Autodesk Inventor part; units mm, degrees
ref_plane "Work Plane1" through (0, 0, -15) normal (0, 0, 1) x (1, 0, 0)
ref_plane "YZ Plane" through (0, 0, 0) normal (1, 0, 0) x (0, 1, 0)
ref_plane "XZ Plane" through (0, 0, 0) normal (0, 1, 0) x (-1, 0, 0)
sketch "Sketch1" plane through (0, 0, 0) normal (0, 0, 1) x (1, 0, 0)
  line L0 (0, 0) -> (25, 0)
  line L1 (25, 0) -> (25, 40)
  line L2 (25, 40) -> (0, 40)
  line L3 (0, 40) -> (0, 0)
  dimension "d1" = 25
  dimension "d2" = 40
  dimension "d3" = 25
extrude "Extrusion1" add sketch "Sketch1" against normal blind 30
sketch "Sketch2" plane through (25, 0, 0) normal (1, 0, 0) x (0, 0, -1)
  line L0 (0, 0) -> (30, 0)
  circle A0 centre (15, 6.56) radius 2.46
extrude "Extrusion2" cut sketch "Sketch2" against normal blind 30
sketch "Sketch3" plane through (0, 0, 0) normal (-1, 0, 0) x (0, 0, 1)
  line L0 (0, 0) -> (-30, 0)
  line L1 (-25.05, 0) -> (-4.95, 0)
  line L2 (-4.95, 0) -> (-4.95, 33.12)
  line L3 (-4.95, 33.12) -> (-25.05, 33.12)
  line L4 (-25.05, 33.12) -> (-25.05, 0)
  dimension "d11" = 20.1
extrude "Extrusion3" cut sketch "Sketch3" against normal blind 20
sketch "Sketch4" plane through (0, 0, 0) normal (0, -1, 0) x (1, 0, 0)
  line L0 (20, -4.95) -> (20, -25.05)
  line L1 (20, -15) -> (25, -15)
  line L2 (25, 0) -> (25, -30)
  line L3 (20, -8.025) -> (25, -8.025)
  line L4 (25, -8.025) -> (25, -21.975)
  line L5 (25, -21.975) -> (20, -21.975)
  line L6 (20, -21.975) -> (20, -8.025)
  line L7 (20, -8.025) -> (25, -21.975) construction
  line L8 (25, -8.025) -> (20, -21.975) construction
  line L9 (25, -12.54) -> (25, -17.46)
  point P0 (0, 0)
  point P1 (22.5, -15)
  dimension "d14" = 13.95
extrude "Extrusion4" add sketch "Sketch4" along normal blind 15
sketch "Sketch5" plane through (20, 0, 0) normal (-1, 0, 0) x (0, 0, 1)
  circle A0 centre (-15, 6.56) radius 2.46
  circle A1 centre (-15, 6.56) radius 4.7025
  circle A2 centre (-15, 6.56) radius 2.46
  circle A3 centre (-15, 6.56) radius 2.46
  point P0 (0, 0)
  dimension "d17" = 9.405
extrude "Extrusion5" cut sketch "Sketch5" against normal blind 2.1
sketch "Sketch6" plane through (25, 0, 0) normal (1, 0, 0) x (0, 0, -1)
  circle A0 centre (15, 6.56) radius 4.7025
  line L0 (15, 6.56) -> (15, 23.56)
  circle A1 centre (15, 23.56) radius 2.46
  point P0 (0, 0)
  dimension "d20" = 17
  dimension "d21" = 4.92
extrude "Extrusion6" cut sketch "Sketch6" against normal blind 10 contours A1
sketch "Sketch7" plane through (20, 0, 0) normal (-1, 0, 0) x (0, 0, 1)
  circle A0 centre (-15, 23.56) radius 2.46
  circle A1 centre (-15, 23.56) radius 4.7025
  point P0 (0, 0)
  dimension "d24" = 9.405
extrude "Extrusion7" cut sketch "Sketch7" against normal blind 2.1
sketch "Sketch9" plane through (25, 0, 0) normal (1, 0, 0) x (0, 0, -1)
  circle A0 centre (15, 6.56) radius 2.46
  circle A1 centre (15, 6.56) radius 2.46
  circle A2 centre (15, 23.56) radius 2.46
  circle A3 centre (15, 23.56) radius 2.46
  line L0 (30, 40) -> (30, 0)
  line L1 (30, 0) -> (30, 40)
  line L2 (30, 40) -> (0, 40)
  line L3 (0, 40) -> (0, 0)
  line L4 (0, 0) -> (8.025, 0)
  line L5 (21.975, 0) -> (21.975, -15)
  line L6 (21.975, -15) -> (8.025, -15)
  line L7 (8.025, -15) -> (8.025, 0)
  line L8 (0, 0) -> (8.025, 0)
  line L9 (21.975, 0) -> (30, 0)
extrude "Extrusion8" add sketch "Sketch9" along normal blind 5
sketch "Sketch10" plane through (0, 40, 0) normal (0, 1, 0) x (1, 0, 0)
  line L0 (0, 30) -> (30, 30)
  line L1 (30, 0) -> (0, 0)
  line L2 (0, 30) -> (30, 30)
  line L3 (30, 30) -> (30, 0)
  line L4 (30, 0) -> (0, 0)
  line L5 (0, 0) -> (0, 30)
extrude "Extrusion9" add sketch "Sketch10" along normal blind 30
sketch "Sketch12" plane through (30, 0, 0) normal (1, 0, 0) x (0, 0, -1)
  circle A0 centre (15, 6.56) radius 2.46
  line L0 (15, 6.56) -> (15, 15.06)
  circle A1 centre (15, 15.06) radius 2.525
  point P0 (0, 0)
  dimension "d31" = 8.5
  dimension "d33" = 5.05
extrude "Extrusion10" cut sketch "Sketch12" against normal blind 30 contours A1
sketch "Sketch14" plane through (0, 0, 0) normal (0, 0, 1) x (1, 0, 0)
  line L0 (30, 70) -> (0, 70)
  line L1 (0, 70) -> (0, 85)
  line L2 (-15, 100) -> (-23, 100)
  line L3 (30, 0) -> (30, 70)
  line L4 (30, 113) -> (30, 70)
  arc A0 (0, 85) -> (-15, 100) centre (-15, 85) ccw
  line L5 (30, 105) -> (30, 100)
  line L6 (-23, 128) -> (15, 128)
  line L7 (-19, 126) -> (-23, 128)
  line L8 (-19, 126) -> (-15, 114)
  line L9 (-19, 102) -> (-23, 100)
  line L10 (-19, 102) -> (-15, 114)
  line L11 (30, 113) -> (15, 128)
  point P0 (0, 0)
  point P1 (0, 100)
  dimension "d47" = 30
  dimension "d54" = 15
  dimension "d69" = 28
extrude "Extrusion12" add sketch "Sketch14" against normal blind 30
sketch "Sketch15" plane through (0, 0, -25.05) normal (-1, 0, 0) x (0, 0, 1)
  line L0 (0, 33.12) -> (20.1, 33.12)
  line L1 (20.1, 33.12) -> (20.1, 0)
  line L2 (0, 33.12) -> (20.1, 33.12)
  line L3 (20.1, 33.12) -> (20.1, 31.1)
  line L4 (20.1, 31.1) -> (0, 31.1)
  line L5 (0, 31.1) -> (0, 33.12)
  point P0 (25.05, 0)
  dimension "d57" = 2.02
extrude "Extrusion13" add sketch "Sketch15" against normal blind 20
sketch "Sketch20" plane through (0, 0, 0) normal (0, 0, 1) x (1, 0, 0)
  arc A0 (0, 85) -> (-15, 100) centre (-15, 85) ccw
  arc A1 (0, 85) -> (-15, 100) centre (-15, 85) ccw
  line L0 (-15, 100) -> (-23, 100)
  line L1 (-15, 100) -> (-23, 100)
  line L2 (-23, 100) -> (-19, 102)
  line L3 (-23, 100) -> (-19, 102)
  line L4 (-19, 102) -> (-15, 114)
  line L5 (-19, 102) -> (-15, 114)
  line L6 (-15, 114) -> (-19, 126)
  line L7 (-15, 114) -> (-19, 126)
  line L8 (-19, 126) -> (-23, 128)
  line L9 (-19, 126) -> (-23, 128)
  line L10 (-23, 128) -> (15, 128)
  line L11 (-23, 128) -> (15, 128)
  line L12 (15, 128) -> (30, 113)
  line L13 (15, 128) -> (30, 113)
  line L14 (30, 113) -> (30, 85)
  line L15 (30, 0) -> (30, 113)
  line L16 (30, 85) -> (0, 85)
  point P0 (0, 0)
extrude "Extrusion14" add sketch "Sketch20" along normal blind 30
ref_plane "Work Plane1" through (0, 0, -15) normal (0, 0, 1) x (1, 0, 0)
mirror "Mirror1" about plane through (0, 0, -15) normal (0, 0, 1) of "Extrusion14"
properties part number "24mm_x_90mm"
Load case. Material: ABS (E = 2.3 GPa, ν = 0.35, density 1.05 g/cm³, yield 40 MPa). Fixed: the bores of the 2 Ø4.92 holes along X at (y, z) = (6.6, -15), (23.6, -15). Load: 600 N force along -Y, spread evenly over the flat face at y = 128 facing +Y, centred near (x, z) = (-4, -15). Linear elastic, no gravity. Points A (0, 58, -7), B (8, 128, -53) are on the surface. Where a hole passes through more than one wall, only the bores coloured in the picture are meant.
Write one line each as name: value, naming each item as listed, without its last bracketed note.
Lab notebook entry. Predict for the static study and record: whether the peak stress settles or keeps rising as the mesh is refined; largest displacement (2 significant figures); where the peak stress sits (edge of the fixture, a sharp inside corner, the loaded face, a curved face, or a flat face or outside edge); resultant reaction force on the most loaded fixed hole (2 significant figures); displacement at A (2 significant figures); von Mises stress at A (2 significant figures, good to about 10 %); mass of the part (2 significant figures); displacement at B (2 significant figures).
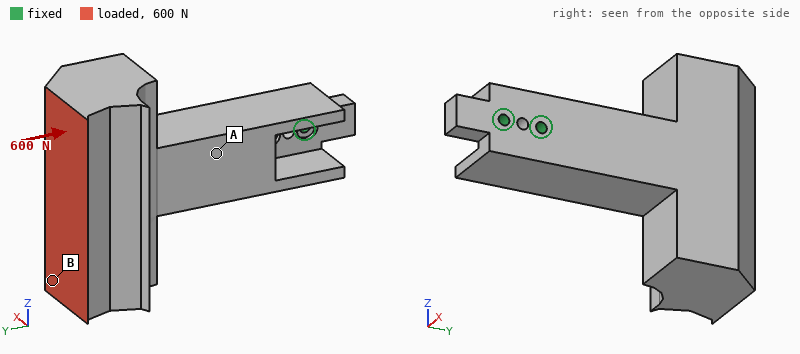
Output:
whether the peak stress settles or keeps rising as the mesh is refined: keeps rising
largest displacement: 1.7 mm
where the peak stress sits: edge of the fixture
resultant reaction force on the most loaded fixed hole: 810 N
displacement at A: 0.55 mm
von Mises stress at A: 3.2 MPa
mass of the part: 230 g
displacement at B: 1.5 mm
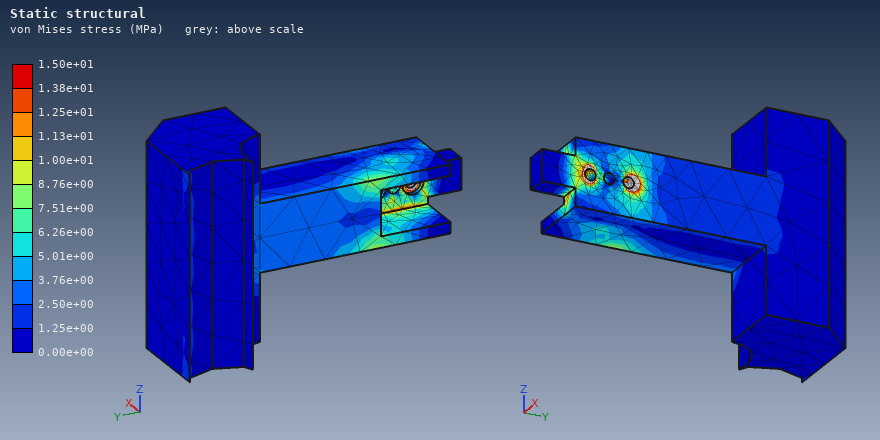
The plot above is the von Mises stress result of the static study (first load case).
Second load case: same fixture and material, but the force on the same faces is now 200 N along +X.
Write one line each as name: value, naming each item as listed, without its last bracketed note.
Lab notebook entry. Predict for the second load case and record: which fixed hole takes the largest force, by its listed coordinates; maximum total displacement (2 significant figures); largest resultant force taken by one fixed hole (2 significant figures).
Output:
which fixed hole takes the largest force, by its listed coordinates: (23.6, -15)
maximum total displacement: 2.1 mm
largest resultant force taken by one fixed hole: 1.0 kN
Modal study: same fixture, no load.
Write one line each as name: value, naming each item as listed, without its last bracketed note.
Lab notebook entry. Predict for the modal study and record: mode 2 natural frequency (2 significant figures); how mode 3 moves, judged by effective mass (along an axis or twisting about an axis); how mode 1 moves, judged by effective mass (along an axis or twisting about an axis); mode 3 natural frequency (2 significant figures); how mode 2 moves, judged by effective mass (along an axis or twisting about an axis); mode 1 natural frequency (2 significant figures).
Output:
mode 2 natural frequency: 170 Hz
how mode 3 moves, judged by effective mass: twisting about Y
how mode 1 moves, judged by effective mass: along X
mode 3 natural frequency: 300 Hz
how mode 2 moves, judged by effective mass: along Z
mode 1 natural frequency: 150 Hz
